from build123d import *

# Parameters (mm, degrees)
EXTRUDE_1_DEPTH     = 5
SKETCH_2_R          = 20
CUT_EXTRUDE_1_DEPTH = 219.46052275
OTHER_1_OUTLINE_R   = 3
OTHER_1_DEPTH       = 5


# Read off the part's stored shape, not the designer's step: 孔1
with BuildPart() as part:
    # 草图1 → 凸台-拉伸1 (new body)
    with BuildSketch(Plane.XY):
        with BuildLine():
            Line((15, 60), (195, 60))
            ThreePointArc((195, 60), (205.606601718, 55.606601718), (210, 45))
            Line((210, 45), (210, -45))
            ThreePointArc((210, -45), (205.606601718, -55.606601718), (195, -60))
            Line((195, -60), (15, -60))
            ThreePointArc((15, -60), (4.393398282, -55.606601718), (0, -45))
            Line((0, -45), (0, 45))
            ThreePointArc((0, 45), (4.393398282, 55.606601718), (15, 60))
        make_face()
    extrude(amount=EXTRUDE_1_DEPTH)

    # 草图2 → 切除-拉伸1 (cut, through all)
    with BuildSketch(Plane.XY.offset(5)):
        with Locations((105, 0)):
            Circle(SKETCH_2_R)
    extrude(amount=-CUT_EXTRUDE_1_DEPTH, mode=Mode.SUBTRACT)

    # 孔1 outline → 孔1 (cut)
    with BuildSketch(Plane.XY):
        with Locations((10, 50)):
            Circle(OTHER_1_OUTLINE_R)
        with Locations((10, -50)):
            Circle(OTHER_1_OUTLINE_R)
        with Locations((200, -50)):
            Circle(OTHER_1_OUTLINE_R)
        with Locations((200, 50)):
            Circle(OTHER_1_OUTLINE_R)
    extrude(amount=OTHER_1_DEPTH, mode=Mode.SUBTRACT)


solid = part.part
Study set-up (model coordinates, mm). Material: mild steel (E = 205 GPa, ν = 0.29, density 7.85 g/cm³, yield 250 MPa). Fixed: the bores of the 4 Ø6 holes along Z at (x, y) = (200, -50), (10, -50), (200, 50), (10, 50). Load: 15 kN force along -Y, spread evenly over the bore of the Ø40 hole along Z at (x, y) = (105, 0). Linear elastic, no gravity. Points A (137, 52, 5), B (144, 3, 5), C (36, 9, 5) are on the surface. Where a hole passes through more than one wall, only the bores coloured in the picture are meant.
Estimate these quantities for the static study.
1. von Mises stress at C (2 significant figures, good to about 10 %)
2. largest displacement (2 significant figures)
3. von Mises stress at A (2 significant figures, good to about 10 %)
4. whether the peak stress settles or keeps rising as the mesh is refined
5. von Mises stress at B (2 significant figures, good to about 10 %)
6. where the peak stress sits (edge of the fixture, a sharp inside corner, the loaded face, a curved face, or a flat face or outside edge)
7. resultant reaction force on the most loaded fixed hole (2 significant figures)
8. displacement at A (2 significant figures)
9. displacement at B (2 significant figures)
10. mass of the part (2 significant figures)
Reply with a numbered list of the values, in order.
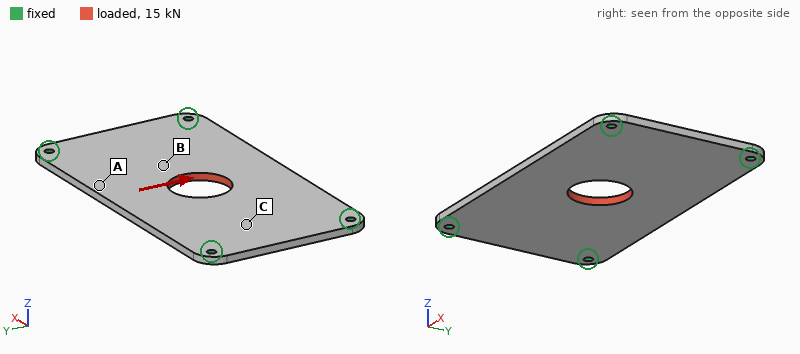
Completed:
1. 27 MPa
2. 23 µm
3. 15 MPa
4. keeps rising
5. 32 MPa
6. edge of the fixture
7. 5.0 kN
8. 17 µm
9. 15 µm
10. 930 g
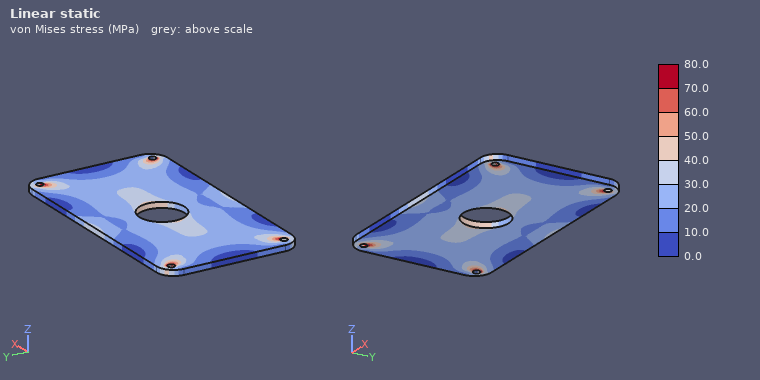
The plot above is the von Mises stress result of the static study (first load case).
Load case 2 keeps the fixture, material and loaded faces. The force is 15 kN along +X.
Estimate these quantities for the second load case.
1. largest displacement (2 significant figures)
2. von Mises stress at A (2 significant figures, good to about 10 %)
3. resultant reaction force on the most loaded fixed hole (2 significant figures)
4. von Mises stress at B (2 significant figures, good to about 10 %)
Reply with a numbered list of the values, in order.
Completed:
1. 11 µm
2. 8.1 MPa
3. 3.9 kN
4. 18 MPa
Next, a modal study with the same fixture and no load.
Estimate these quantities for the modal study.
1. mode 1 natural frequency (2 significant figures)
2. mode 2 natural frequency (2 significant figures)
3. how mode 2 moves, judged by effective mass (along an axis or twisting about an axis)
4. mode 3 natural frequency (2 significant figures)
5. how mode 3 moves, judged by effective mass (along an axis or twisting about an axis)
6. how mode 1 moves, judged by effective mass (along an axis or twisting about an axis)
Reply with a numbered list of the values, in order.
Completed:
1. 620 Hz
2. 1000 Hz
3. twisting about X
4. 1600 Hz
5. twisting about Y
6. along Z
